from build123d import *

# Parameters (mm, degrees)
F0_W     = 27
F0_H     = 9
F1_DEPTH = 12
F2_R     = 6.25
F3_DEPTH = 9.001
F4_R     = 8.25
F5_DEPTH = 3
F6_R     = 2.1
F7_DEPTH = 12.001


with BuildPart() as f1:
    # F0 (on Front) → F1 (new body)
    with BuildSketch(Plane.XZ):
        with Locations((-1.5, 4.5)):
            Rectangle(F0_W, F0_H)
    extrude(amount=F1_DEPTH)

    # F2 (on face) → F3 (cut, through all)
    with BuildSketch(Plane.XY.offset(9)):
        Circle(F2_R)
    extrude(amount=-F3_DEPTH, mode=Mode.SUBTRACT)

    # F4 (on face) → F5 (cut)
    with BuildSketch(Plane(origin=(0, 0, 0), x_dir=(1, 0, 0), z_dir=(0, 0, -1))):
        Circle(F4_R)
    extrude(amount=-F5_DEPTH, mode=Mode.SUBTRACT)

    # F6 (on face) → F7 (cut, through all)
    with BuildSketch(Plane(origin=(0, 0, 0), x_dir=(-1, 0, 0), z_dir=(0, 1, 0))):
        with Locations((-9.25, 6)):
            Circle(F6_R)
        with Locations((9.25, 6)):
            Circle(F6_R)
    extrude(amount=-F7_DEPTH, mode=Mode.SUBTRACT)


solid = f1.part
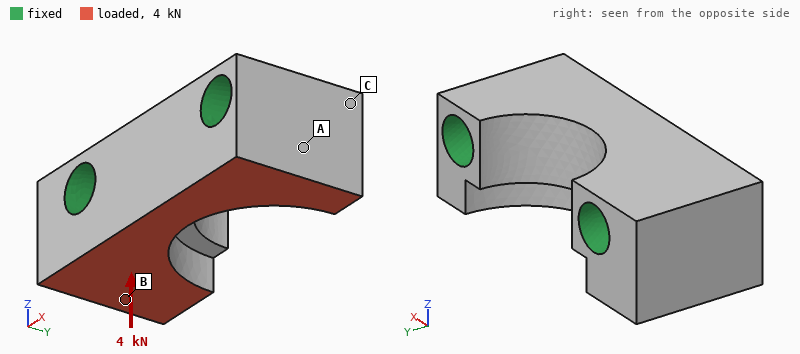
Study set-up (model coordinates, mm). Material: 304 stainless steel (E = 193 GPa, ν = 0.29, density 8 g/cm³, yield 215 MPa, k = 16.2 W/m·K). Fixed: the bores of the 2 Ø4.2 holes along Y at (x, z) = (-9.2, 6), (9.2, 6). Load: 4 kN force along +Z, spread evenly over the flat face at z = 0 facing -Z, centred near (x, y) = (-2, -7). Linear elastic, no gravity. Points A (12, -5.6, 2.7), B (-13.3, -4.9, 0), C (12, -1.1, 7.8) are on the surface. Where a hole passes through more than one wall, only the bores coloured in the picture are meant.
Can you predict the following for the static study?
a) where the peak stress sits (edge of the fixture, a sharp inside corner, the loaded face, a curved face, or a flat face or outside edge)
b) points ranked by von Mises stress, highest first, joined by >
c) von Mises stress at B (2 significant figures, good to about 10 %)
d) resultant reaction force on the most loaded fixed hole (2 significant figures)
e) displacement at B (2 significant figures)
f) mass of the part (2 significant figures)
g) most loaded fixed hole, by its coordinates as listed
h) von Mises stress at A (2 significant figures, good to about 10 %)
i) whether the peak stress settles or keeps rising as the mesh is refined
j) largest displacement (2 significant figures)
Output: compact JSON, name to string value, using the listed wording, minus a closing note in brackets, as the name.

{"where the peak stress sits": "edge of the fixture", "points ranked by von Mises stress, highest first, joined by >": "B > A > C", "von Mises stress at B": "19 MPa", "resultant reaction force on the most loaded fixed hole": "2.4 kN", "displacement at B": "0.91 µm", "mass of the part": "15 g", "most loaded fixed hole, by its coordinates as listed": "(-9.2, 6)", "von Mises stress at A": "11 MPa", "whether the peak stress settles or keeps rising as the mesh is refined": "keeps rising", "largest displacement": "1.7 µm"}
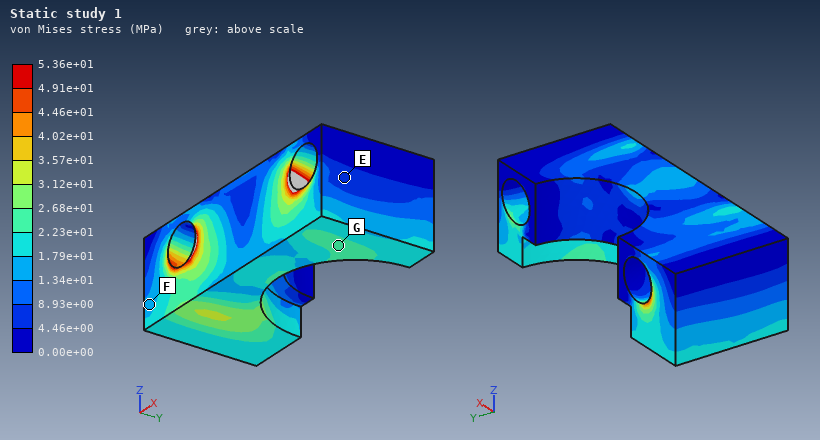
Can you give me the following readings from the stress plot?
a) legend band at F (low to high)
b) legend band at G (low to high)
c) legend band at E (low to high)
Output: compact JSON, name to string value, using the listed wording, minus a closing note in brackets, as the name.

{"legend band at F": "1.34e+01 to 1.79e+01 MPa", "legend band at G": "2.23e+01 to 2.68e+01 MPa", "legend band at E": "4.46e+00 to 8.93e+00 MPa"}
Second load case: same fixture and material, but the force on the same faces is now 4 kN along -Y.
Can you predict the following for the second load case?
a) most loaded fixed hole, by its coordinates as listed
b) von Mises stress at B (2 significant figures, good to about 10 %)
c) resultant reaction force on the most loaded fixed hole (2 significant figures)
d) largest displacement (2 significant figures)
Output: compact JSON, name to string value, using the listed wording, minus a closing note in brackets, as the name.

{"most loaded fixed hole, by its coordinates as listed": "(-9.2, 6)", "von Mises stress at B": "34 MPa", "resultant reaction force on the most loaded fixed hole": "2.3 kN", "largest displacement": "4.9 µm"}
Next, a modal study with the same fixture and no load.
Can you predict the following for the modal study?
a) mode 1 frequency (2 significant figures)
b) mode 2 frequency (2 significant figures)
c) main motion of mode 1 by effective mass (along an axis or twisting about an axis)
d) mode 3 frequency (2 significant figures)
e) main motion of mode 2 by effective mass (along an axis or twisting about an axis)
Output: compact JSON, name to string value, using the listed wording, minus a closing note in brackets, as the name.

{"mode 1 frequency": "75 kHz", "mode 2 frequency": "88 kHz", "main motion of mode 1 by effective mass": "along Z", "mode 3 frequency": "98 kHz", "main motion of mode 2 by effective mass": "along Y"}
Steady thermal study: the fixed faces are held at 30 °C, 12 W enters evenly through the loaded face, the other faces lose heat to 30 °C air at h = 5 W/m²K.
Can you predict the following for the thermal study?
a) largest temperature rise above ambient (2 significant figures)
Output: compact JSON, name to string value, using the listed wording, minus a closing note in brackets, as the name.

{"largest temperature rise above ambient": "23 K"}
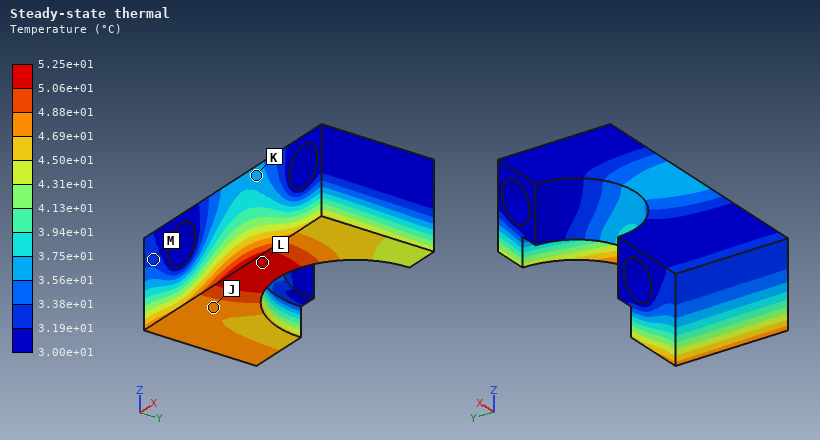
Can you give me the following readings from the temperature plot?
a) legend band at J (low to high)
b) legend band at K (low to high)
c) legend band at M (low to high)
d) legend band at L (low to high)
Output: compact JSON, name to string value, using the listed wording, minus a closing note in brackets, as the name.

{"legend band at J": "4.69e+01 to 4.88e+01 °C", "legend band at K": "3.56e+01 to 3.75e+01 °C", "legend band at M": "3.19e+01 to 3.38e+01 °C", "legend band at L": "5.06e+01 to 5.25e+01 °C"}
